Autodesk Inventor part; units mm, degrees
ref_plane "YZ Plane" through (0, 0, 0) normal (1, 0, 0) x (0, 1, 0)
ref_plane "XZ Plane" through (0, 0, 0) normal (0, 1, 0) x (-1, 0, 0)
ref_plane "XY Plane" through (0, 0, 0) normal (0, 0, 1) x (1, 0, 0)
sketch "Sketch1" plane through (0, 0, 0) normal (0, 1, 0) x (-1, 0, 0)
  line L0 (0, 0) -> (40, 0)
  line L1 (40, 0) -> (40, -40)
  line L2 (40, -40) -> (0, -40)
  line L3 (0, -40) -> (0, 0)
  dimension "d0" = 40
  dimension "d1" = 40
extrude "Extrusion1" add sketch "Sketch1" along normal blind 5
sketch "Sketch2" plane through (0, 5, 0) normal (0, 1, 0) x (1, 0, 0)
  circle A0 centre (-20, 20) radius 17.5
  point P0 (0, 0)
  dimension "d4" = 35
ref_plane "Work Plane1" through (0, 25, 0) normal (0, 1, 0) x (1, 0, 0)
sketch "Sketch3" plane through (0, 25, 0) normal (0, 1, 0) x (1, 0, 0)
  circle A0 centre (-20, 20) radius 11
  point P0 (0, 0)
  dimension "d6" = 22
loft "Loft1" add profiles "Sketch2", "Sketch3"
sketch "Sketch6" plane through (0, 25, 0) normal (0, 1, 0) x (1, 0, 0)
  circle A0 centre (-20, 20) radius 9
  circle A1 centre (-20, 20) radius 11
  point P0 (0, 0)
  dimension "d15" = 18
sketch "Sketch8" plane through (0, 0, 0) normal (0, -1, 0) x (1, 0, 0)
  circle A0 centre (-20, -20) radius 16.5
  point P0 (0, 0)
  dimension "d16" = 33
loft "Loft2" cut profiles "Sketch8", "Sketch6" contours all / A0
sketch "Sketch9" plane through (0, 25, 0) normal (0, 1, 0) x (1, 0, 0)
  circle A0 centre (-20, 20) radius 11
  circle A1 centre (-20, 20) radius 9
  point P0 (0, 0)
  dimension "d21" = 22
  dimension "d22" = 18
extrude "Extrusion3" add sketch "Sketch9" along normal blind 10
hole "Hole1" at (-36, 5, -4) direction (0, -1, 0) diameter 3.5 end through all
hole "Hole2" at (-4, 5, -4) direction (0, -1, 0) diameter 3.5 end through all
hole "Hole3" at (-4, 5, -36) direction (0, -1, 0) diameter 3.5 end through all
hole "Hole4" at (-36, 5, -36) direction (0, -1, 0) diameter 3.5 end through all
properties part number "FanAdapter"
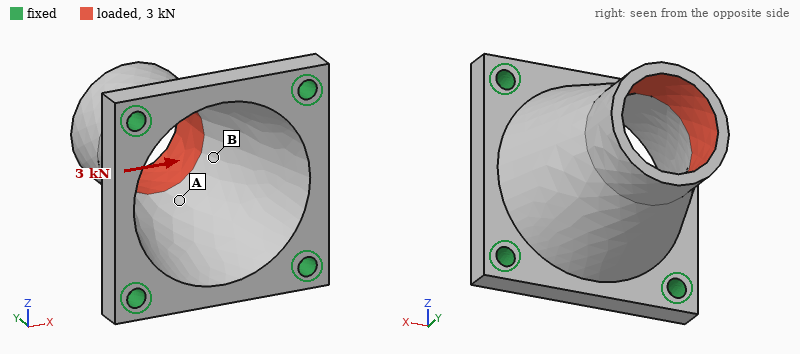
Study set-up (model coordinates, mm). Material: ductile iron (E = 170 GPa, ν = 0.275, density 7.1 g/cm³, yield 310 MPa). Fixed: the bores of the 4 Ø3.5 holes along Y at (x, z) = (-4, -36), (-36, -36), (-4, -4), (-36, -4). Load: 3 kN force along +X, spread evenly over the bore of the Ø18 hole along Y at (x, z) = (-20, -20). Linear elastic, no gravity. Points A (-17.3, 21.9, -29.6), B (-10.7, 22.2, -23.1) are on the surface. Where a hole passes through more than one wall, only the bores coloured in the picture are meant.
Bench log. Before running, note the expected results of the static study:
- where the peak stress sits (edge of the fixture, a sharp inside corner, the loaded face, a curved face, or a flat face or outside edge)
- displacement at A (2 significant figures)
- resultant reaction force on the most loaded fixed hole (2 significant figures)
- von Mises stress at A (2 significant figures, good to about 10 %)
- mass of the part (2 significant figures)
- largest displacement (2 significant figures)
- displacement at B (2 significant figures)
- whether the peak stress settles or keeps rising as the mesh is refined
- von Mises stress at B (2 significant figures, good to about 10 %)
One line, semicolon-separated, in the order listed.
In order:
edge of the fixture; 16 µm; 1.7 kN; 72 MPa; 63 g; 34 µm; 19 µm; keeps rising; 22 MPa
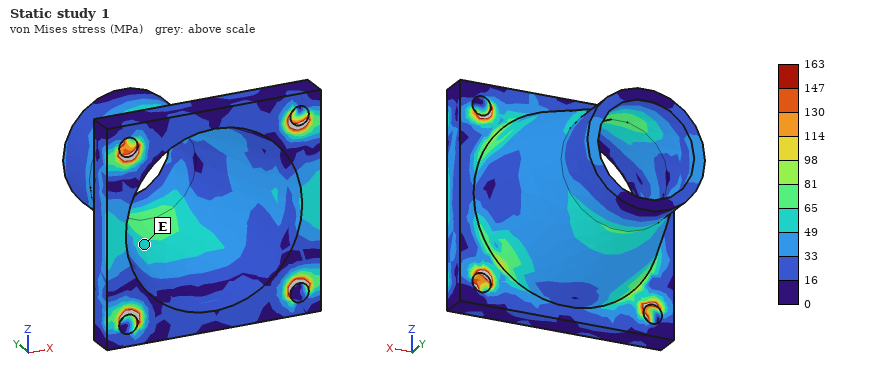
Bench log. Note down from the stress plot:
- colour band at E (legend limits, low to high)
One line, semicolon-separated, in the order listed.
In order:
49 to 65 MPa
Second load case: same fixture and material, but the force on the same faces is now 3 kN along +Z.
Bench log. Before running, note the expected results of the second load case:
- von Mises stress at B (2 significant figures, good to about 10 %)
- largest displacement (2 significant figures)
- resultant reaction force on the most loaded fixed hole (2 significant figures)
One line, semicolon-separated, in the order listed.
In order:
71 MPa; 34 µm; 1.7 kN
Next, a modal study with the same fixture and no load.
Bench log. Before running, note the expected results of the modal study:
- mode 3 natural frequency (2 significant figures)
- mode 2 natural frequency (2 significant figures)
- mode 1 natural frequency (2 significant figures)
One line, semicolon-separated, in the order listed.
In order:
13 kHz; 13 kHz; 13 kHz
